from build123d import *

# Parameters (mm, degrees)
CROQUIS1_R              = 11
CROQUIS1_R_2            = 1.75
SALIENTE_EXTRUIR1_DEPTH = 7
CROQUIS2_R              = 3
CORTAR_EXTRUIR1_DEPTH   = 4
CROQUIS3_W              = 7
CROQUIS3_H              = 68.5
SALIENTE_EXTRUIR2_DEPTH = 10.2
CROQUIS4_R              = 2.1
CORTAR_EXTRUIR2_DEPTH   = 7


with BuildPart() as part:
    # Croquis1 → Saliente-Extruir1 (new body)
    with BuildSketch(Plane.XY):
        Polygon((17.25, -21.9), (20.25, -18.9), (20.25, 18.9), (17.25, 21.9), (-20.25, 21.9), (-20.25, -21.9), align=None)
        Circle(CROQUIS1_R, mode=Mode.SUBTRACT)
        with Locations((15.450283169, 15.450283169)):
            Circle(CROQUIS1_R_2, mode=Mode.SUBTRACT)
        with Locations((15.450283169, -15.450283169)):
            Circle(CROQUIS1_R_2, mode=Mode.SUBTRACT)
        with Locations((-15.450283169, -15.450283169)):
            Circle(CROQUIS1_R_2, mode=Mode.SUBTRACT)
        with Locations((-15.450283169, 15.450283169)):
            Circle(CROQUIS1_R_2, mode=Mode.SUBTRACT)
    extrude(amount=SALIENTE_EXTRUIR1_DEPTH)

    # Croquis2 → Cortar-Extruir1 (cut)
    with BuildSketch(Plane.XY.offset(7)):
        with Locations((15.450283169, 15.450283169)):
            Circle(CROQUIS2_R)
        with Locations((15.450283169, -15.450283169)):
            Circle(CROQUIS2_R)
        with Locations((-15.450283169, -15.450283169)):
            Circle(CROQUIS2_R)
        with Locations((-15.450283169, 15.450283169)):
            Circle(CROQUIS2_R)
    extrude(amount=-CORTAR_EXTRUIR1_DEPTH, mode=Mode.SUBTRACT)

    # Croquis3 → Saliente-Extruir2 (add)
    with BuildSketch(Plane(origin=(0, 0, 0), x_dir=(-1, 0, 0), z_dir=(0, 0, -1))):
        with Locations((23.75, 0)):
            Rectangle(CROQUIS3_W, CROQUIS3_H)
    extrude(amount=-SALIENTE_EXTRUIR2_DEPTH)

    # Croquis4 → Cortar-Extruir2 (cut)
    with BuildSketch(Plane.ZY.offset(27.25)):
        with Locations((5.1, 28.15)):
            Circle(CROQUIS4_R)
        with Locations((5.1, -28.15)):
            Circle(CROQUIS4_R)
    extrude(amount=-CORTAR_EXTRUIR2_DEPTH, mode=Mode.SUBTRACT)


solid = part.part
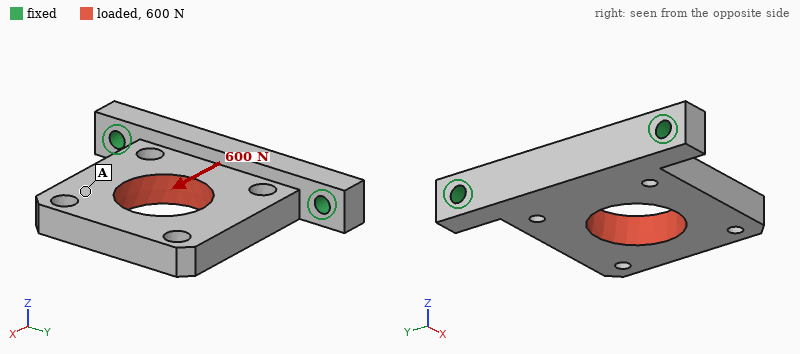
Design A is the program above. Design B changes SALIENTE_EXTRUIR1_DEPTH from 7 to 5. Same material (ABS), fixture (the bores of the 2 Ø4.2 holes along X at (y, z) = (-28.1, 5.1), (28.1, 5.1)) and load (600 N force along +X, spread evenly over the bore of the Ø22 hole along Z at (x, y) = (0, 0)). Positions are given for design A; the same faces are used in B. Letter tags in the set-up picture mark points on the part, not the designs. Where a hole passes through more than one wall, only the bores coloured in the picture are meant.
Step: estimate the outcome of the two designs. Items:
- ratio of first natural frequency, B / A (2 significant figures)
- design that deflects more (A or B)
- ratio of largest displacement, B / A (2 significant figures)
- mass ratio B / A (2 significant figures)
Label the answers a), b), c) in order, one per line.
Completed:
a) 0.90
b) B
c) 1.7
d) 0.82
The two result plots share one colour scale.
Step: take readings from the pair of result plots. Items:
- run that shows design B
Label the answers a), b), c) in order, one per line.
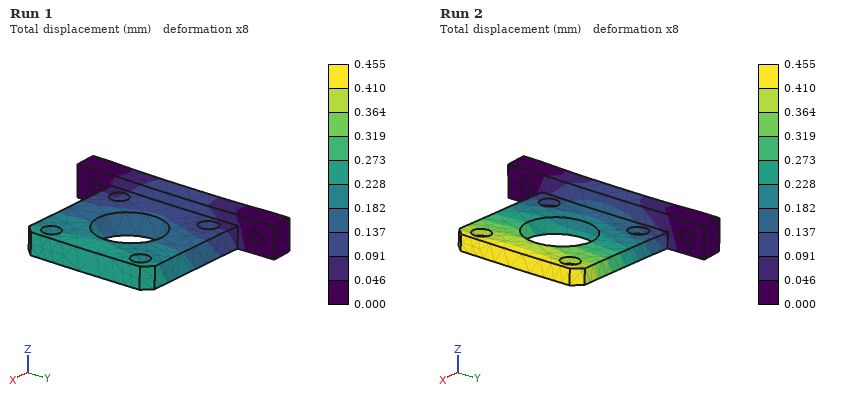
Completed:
a) Run 2
